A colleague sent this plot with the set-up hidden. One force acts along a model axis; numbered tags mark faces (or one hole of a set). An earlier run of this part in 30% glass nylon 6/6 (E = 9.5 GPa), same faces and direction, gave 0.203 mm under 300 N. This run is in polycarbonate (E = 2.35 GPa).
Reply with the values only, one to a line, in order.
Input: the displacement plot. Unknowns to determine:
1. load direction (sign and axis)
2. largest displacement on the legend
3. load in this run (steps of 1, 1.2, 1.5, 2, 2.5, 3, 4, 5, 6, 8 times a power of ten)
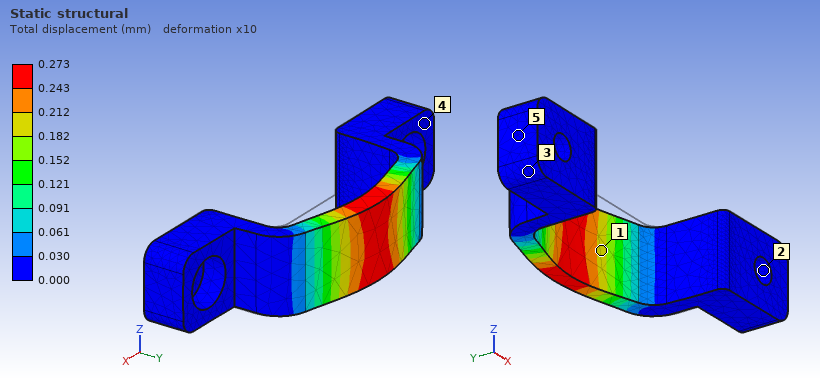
+Y
0.273 mm
100 N
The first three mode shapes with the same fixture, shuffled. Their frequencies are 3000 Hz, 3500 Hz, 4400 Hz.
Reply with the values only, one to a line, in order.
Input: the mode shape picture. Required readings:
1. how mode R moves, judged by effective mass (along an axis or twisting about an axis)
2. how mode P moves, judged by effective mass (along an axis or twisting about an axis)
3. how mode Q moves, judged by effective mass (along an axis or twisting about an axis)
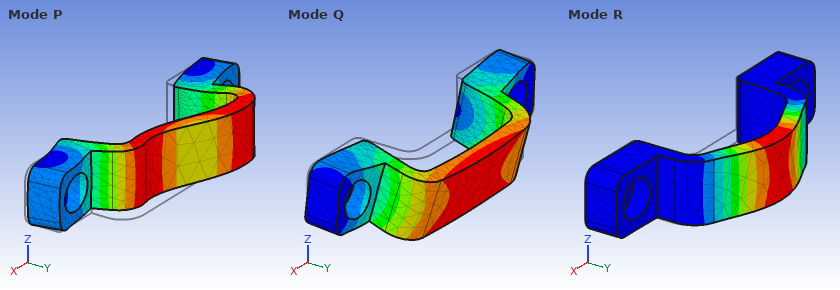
along Y
along X
along Z
